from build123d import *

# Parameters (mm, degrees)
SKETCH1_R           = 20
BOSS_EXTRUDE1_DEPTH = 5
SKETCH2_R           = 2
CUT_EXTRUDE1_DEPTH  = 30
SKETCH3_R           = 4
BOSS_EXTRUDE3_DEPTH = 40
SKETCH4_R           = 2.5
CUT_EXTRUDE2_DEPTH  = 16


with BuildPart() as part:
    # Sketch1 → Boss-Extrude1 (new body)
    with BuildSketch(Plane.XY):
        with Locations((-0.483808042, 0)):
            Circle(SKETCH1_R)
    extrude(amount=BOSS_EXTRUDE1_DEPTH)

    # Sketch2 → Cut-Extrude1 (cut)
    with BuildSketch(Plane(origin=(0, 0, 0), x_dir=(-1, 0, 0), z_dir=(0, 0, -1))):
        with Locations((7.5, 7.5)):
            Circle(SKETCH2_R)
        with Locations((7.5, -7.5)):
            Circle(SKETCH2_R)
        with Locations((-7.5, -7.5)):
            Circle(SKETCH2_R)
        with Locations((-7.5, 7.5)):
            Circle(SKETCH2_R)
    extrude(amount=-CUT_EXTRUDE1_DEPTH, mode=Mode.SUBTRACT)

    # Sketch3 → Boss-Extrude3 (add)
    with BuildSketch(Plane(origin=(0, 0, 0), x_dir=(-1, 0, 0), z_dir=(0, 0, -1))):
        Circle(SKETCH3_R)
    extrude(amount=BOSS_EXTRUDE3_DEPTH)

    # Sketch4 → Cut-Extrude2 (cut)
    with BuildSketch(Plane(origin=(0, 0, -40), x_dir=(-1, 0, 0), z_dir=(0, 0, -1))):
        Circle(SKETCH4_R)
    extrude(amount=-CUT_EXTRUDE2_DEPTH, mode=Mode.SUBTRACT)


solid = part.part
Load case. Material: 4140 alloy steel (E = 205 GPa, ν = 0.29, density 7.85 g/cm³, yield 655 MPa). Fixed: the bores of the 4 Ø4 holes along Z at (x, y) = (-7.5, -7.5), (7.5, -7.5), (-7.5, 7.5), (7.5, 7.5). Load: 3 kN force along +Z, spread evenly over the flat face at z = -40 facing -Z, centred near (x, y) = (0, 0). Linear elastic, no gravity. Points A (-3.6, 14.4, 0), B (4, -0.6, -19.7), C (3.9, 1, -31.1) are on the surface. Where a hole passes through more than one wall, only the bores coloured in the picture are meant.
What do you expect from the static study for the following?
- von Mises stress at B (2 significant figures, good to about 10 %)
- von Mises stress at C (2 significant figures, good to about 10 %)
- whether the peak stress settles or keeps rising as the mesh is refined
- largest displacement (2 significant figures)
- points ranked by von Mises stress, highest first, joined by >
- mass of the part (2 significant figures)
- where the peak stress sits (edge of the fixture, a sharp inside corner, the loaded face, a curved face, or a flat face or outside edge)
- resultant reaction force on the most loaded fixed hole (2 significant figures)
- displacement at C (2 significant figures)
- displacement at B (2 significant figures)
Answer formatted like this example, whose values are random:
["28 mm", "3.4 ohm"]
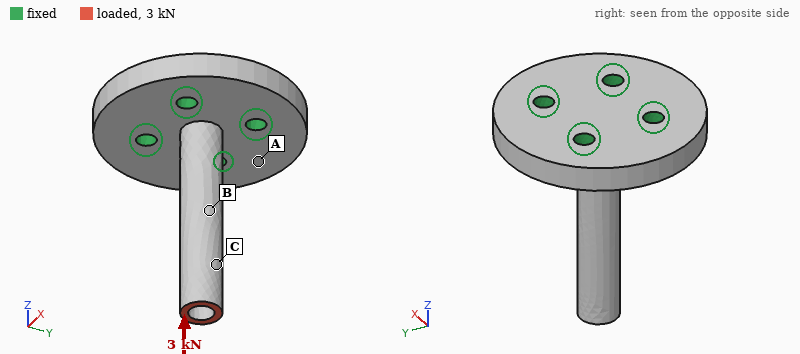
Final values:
["64 MPa", "98 MPa", "keeps rising", "18 µm", "C > B > A", "61 g", "edge of the fixture", "770 N", "14 µm", "8.6 µm"]
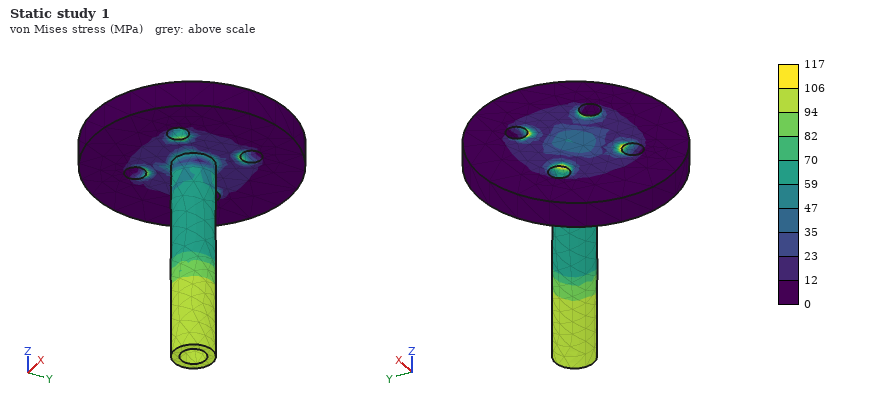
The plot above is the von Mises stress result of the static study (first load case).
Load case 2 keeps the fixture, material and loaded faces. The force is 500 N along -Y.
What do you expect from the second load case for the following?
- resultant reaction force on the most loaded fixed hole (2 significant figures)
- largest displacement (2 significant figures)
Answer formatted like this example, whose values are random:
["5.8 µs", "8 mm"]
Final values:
["850 N", "0.32 mm"]
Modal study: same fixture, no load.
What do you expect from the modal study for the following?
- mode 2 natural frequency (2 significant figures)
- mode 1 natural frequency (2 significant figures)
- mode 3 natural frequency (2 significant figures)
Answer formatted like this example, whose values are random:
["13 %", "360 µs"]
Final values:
["3800 Hz", "3800 Hz", "19 kHz"]
